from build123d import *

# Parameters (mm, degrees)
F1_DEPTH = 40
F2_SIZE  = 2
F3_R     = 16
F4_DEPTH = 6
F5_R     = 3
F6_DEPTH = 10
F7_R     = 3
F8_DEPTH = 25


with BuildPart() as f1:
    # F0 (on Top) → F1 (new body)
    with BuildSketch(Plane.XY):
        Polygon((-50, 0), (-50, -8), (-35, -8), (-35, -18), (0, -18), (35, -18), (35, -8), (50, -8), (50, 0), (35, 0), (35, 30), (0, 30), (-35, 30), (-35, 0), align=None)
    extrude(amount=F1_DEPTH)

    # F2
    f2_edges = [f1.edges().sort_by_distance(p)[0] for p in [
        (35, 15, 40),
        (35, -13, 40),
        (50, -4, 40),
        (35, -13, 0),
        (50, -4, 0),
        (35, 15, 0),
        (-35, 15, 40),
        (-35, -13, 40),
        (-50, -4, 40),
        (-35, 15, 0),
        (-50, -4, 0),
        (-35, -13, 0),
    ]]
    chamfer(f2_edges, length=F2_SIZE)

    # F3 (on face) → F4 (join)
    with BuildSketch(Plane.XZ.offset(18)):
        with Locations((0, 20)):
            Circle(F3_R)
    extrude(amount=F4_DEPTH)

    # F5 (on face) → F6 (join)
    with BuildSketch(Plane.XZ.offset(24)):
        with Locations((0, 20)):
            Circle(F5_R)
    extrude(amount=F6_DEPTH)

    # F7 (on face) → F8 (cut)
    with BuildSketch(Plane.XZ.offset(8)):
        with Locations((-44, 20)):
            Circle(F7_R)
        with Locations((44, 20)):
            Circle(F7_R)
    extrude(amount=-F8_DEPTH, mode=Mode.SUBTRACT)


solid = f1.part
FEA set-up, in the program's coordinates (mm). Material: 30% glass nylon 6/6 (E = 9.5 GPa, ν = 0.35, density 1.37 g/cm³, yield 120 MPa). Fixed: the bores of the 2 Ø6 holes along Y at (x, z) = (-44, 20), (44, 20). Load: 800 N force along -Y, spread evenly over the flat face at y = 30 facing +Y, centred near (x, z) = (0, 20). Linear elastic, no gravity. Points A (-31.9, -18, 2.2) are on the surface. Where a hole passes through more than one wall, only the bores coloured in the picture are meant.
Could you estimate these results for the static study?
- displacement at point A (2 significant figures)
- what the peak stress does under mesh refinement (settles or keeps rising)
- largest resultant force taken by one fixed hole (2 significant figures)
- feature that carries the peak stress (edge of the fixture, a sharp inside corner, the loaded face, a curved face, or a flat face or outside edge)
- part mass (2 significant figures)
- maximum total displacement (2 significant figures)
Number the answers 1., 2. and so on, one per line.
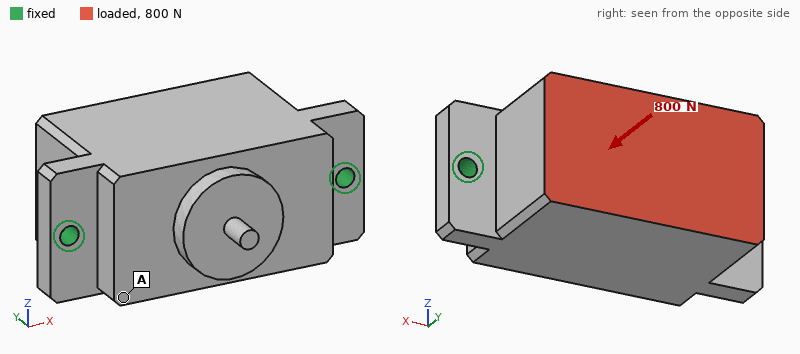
1. 13 µm
2. keeps rising
3. 400 N
4. edge of the fixture
5. 200 g
6. 15 µm
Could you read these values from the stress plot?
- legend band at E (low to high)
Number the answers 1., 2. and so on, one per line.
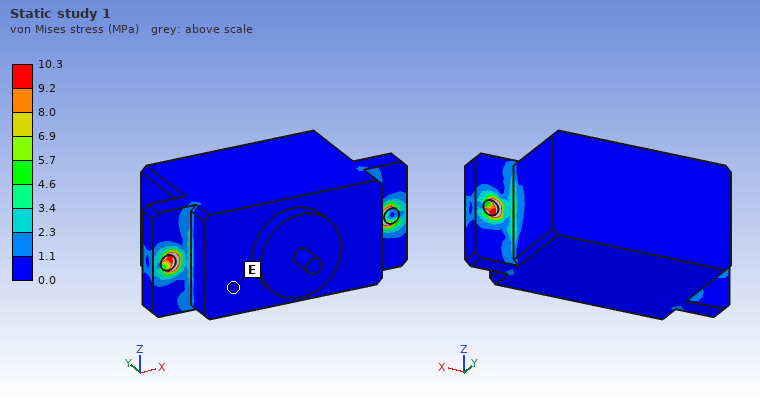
1. 0.0 to 1.1 MPa
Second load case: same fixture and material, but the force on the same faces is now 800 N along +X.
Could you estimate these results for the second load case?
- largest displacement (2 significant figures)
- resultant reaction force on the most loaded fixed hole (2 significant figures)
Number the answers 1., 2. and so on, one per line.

1. 20 µm
2. 530 N
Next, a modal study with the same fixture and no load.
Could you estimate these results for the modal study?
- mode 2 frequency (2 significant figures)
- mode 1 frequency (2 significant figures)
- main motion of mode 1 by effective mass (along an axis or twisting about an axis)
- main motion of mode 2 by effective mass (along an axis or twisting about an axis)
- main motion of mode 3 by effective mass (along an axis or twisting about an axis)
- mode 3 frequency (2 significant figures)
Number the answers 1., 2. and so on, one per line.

1. 2800 Hz
2. 1100 Hz
3. along Z
4. along Y
5. along Z
6. 3600 Hz
